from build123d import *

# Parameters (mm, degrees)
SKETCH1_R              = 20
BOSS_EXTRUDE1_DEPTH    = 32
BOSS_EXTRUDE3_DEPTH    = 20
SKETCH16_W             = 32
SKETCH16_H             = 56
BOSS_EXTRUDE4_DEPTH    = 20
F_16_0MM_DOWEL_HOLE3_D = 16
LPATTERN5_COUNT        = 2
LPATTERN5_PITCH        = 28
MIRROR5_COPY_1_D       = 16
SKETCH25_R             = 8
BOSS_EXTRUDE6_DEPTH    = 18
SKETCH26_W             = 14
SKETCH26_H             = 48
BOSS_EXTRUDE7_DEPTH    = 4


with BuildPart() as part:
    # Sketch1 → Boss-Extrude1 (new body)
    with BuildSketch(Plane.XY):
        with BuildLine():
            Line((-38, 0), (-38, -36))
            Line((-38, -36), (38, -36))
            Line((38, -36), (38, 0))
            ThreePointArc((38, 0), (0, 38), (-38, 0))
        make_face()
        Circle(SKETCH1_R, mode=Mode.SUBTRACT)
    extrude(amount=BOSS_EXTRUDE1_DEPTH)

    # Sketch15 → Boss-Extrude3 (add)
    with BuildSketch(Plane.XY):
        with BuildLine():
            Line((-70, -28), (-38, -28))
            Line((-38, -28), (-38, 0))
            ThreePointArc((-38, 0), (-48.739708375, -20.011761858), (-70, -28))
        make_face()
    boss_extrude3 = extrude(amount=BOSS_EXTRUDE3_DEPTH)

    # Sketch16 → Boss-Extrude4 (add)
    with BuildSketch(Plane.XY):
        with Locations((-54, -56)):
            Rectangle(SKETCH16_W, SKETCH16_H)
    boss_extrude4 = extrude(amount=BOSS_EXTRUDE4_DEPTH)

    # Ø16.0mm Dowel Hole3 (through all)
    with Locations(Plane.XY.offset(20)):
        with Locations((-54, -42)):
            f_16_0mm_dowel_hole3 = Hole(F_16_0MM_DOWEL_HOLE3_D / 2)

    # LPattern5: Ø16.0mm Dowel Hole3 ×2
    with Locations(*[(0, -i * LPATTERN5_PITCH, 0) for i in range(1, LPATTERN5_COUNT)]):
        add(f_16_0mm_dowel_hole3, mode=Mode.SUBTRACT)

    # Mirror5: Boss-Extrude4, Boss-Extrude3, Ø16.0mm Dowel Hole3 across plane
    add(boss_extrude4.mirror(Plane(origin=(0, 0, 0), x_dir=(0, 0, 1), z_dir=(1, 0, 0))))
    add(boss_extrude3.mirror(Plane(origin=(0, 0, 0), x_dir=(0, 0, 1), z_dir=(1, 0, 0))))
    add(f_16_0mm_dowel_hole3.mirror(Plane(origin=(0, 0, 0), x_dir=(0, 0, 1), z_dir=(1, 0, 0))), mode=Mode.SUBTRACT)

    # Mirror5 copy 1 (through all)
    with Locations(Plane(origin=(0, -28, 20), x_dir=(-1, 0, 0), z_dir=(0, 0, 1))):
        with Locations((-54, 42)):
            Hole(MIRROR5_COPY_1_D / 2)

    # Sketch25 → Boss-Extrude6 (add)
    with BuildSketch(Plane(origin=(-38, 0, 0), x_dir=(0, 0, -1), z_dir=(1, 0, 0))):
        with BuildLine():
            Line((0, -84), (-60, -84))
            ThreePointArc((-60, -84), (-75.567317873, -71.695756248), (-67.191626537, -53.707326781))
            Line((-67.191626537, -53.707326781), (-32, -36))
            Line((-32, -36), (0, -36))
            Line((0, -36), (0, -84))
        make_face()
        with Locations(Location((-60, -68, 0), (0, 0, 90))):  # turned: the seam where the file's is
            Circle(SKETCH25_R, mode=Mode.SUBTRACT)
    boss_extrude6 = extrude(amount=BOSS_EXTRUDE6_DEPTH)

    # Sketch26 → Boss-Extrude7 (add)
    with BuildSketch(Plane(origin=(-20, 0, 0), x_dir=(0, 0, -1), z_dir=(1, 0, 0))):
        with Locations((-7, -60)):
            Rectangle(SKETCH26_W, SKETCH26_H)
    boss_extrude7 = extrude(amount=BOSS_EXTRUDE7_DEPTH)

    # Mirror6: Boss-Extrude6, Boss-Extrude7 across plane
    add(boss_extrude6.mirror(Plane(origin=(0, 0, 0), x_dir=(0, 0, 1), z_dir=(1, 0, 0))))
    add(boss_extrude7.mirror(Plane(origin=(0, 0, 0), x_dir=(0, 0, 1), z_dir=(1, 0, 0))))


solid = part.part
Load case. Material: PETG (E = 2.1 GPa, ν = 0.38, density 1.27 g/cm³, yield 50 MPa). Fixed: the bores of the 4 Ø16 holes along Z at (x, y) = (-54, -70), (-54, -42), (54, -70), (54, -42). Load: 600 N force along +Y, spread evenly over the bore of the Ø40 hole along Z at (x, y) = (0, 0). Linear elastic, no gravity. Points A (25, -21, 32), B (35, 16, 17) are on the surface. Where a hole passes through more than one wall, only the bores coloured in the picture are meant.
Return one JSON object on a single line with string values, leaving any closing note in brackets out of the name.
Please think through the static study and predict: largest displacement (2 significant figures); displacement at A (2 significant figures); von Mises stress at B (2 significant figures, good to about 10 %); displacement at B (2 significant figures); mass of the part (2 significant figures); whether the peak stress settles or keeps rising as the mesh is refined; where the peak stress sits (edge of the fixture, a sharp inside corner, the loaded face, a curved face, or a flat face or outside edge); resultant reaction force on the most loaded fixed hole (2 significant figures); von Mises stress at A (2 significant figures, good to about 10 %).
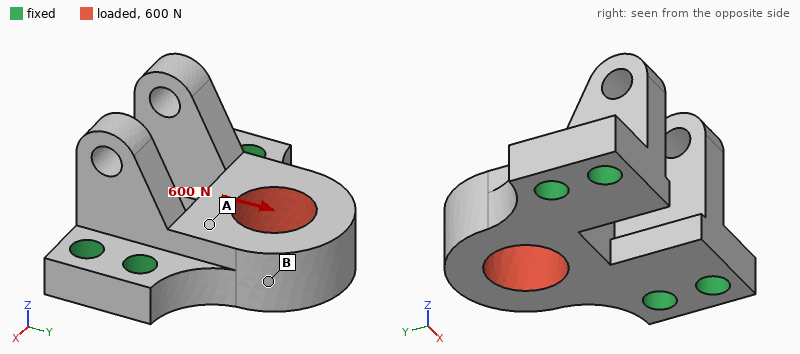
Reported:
{"largest displacement": "33 µm", "displacement at A": "16 µm", "von Mises stress at B": "0.13 MPa", "displacement at B": "21 µm", "mass of the part": "370 g", "whether the peak stress settles or keeps rising as the mesh is refined": "keeps rising", "where the peak stress sits": "edge of the fixture", "resultant reaction force on the most loaded fixed hole": "200 N", "von Mises stress at A": "0.36 MPa"}
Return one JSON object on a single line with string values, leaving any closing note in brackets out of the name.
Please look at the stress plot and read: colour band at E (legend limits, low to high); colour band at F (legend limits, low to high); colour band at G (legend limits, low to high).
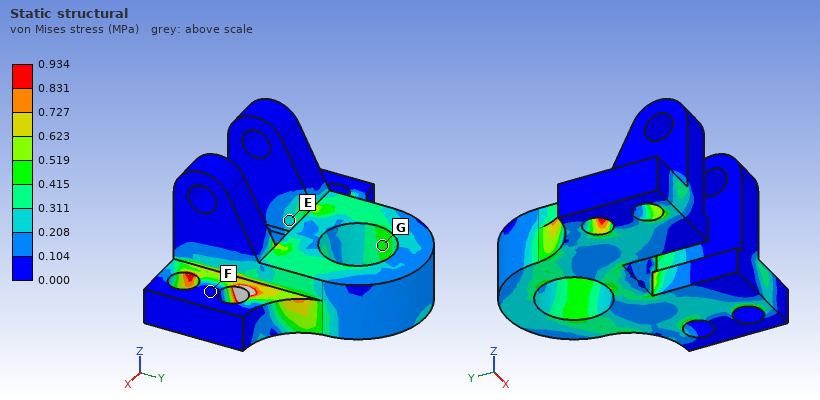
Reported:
{"colour band at E": "0.208 to 0.311 MPa", "colour band at F": "0.000 to 0.104 MPa", "colour band at G": "0.415 to 0.519 MPa"}
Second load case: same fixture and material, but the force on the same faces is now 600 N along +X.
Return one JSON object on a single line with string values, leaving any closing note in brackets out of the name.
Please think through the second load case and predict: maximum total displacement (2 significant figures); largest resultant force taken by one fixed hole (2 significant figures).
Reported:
{"maximum total displacement": "47 µm", "largest resultant force taken by one fixed hole": "360 N"}
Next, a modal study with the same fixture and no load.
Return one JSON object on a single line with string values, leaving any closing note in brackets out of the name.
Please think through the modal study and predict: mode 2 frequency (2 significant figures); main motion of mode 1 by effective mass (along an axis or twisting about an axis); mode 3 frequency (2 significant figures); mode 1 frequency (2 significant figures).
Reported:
{"mode 2 frequency": "1100 Hz", "main motion of mode 1 by effective mass": "along Z", "mode 3 frequency": "1100 Hz", "mode 1 frequency": "750 Hz"}
